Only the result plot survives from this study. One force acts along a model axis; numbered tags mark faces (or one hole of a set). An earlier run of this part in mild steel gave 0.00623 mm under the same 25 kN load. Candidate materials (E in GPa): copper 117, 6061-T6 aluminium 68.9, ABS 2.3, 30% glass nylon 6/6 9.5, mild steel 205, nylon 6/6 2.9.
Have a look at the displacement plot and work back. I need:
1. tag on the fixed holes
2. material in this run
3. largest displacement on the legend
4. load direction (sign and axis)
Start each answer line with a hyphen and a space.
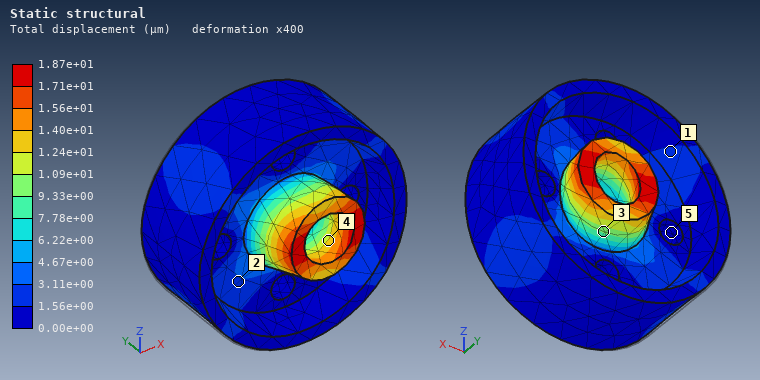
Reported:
- 5
- 6061-T6 aluminium
- 1.87e+01 µm
- +X
